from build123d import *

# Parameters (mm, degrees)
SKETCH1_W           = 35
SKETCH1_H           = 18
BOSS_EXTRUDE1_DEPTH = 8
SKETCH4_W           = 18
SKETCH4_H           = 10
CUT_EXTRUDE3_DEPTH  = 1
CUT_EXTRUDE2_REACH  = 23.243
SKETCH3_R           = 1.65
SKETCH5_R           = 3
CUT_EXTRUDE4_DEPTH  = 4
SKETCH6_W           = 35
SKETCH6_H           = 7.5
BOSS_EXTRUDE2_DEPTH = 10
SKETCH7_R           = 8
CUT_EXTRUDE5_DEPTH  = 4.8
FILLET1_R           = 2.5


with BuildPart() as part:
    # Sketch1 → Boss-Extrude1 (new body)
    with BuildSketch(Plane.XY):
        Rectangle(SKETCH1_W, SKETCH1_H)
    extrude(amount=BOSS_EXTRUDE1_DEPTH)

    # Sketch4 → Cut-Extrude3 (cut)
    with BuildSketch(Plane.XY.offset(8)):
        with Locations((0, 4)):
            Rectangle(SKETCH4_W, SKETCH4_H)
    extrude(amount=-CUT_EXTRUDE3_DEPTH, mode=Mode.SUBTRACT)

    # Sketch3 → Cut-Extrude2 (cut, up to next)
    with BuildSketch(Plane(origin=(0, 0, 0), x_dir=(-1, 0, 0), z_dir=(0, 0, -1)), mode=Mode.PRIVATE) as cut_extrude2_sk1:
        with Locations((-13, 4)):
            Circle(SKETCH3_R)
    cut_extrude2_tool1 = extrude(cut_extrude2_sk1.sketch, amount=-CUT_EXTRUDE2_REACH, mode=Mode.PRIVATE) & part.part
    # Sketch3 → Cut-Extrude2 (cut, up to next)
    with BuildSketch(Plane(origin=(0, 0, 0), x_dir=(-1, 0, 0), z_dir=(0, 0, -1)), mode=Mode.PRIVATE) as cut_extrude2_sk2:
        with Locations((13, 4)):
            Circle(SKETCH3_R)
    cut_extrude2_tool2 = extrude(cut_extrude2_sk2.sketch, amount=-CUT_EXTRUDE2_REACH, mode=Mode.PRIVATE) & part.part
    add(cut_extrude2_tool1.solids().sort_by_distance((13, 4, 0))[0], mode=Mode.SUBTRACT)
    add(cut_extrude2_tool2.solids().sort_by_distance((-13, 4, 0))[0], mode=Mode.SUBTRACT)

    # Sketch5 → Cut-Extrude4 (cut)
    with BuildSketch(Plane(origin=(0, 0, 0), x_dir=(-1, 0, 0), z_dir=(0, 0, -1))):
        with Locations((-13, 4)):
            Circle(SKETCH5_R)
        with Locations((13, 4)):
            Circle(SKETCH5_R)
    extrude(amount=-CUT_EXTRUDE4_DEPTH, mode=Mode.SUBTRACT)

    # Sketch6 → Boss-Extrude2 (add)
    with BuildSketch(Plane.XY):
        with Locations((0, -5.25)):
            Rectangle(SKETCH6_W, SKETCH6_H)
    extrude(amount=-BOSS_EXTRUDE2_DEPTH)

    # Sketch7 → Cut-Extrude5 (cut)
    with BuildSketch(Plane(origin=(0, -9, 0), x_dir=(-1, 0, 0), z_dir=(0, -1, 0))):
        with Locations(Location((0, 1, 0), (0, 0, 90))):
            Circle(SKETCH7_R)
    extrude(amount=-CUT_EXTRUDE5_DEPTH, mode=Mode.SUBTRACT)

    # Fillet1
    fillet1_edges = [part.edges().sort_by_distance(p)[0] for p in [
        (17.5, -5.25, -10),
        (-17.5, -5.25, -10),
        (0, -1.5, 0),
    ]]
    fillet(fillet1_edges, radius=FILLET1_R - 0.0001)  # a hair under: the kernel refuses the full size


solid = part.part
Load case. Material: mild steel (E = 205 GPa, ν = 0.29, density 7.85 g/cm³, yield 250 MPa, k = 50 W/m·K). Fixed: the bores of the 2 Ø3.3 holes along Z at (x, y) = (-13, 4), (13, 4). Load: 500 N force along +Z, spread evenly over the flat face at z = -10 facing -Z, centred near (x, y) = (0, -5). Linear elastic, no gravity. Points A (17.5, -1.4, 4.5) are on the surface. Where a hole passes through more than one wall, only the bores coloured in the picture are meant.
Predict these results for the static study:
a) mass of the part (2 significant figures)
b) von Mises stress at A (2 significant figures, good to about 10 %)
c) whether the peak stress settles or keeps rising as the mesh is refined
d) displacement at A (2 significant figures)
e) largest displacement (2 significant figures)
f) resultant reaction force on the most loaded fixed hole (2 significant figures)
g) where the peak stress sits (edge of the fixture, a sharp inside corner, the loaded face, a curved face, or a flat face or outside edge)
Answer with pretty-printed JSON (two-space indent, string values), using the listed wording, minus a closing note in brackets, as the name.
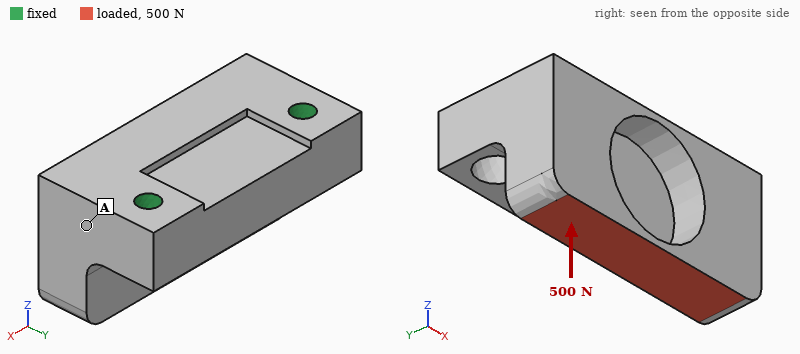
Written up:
{
  "mass of the part": "49 g",
  "von Mises stress at A": "8.1 MPa",
  "whether the peak stress settles or keeps rising as the mesh is refined": "keeps rising",
  "displacement at A": "1.5 µm",
  "largest displacement": "8.2 µm",
  "resultant reaction force on the most loaded fixed hole": "250 N",
  "where the peak stress sits": "edge of the fixture"
}
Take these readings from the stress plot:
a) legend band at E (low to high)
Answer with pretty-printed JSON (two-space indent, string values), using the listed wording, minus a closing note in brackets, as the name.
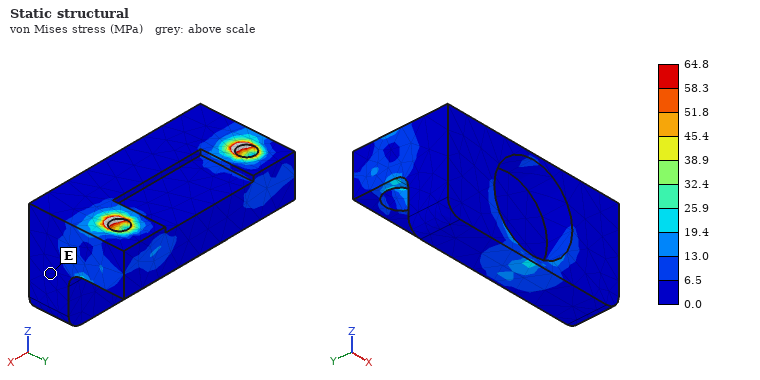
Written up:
{
  "legend band at E": "0.0 to 6.5 MPa"
}
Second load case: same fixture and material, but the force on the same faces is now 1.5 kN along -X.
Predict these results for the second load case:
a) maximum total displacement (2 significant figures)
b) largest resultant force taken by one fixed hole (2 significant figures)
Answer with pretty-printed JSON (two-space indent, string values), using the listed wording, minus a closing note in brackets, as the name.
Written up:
{
  "maximum total displacement": "6.0 µm",
  "largest resultant force taken by one fixed hole": "1.2 kN"
}
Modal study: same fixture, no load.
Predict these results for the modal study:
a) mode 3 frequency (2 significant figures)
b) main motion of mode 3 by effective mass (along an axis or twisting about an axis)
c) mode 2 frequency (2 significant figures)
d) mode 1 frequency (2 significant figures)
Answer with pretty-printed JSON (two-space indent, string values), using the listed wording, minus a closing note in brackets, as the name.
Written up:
{
  "mode 3 frequency": "24 kHz",
  "main motion of mode 3 by effective mass": "along X",
  "mode 2 frequency": "15 kHz",
  "mode 1 frequency": "8200 Hz"
}
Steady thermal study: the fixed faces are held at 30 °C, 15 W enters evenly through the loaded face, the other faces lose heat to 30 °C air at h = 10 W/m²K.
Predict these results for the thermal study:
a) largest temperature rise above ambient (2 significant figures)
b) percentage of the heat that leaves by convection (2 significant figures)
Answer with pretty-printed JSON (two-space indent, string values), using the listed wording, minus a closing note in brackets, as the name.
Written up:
{
  "largest temperature rise above ambient": "44 K",
  "percentage of the heat that leaves by convection": "3.1 %"
}
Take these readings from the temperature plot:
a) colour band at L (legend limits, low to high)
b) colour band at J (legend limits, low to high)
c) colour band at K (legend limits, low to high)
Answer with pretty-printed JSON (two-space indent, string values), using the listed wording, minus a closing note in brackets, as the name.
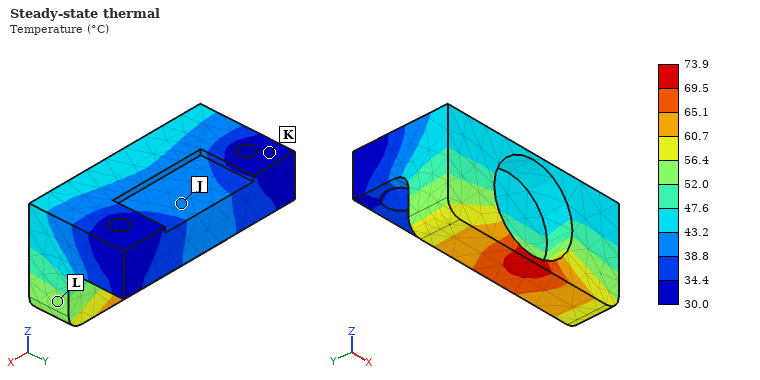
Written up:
{
  "colour band at L": "52.0 to 56.4 °C",
  "colour band at J": "38.8 to 43.2 °C",
  "colour band at K": "30.0 to 34.4 °C"
}
